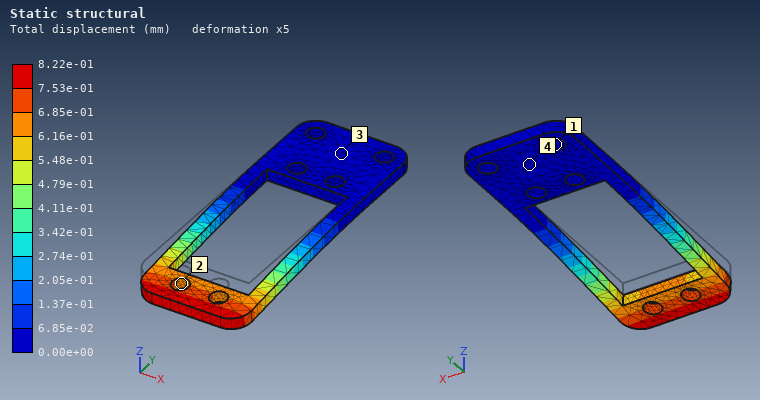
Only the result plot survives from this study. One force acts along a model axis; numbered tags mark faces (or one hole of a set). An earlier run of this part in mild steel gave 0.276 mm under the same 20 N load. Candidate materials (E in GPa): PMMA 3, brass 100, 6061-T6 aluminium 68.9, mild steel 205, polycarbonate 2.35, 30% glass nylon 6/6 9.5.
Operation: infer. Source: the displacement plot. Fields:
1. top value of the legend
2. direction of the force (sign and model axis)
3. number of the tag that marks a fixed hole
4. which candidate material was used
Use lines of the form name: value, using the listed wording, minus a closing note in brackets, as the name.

top value of the legend: 8.22e-01 mm
direction of the force: -Z
number of the tag that marks a fixed hole: 1
which candidate material was used: 6061-T6 aluminium
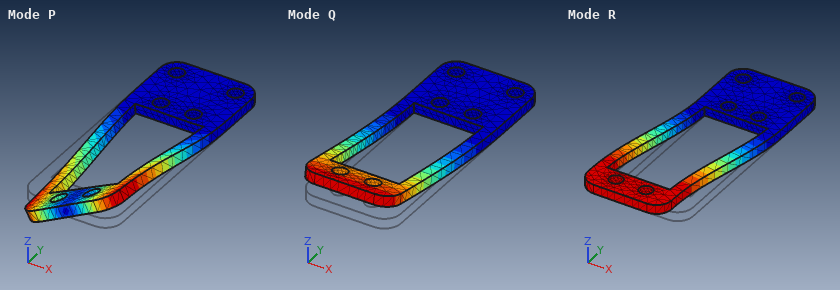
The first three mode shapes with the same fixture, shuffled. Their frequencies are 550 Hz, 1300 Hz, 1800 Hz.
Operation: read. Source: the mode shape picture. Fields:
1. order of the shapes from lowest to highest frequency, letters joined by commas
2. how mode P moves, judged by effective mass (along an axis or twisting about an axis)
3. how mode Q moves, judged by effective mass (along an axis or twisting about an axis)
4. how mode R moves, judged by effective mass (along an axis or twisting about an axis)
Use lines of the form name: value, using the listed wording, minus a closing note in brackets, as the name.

order of the shapes from lowest to highest frequency, letters joined by commas: Q, R, P
how mode P moves, judged by effective mass: twisting about Y
how mode Q moves, judged by effective mass: along Z
how mode R moves, judged by effective mass: along X
